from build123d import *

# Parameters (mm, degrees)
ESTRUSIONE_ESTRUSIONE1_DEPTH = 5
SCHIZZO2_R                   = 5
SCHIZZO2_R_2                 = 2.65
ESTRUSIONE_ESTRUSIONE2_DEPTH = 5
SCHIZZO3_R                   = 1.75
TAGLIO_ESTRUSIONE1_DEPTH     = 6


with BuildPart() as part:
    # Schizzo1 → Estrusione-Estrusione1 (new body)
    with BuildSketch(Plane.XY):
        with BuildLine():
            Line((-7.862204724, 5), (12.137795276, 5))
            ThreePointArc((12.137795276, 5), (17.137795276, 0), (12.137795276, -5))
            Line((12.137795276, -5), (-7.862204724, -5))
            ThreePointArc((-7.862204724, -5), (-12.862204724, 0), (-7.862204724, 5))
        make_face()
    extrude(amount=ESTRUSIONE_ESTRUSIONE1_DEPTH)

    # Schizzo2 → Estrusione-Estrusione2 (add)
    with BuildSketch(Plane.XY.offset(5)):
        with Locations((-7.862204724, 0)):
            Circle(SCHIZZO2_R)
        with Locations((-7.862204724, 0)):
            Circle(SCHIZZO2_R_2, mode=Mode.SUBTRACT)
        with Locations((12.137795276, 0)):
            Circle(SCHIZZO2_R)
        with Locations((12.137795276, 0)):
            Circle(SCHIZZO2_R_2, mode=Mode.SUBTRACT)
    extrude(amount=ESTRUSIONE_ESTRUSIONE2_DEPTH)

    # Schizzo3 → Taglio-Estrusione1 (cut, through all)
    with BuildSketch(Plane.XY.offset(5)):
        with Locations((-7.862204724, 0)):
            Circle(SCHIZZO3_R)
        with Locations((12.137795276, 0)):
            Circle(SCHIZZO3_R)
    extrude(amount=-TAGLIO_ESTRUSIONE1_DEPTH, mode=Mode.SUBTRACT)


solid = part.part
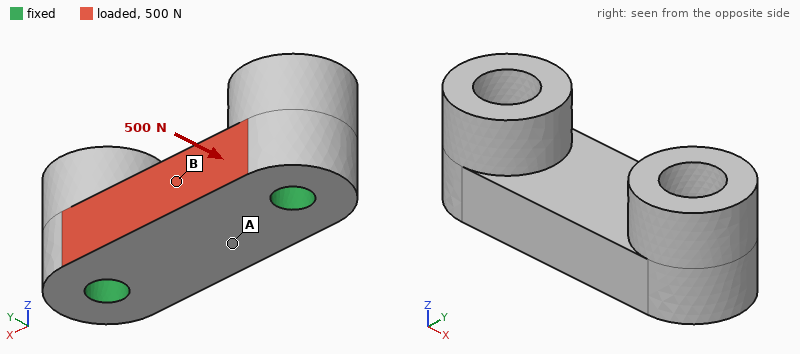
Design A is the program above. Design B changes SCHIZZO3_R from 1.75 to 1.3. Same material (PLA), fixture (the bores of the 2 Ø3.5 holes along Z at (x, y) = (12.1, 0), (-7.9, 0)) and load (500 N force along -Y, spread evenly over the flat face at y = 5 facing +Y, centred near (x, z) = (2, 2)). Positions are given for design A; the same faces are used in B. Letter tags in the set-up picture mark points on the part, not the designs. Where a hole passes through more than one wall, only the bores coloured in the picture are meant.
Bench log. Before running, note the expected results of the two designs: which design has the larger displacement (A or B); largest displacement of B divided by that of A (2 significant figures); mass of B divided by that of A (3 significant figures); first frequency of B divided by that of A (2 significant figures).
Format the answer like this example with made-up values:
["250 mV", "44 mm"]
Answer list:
["B", "1.2", "1.02", "0.87"]
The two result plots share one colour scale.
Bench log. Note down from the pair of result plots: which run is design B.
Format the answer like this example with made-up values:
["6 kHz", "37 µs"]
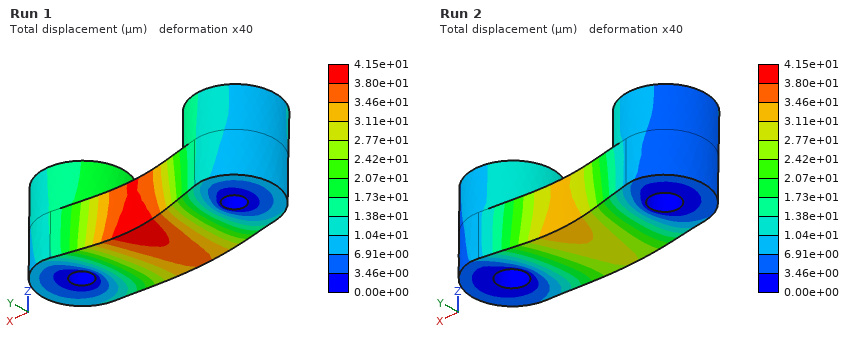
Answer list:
["Run 1"]
